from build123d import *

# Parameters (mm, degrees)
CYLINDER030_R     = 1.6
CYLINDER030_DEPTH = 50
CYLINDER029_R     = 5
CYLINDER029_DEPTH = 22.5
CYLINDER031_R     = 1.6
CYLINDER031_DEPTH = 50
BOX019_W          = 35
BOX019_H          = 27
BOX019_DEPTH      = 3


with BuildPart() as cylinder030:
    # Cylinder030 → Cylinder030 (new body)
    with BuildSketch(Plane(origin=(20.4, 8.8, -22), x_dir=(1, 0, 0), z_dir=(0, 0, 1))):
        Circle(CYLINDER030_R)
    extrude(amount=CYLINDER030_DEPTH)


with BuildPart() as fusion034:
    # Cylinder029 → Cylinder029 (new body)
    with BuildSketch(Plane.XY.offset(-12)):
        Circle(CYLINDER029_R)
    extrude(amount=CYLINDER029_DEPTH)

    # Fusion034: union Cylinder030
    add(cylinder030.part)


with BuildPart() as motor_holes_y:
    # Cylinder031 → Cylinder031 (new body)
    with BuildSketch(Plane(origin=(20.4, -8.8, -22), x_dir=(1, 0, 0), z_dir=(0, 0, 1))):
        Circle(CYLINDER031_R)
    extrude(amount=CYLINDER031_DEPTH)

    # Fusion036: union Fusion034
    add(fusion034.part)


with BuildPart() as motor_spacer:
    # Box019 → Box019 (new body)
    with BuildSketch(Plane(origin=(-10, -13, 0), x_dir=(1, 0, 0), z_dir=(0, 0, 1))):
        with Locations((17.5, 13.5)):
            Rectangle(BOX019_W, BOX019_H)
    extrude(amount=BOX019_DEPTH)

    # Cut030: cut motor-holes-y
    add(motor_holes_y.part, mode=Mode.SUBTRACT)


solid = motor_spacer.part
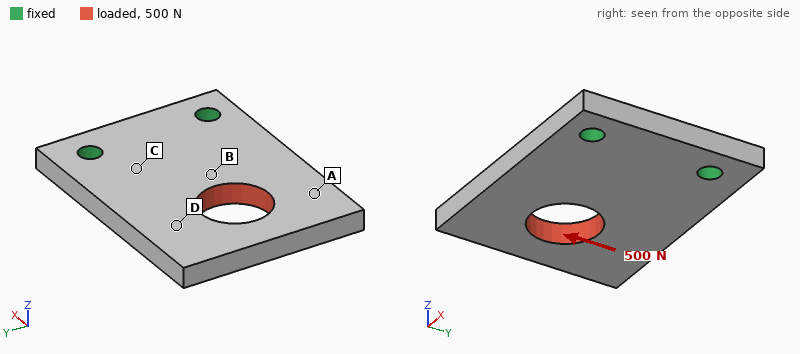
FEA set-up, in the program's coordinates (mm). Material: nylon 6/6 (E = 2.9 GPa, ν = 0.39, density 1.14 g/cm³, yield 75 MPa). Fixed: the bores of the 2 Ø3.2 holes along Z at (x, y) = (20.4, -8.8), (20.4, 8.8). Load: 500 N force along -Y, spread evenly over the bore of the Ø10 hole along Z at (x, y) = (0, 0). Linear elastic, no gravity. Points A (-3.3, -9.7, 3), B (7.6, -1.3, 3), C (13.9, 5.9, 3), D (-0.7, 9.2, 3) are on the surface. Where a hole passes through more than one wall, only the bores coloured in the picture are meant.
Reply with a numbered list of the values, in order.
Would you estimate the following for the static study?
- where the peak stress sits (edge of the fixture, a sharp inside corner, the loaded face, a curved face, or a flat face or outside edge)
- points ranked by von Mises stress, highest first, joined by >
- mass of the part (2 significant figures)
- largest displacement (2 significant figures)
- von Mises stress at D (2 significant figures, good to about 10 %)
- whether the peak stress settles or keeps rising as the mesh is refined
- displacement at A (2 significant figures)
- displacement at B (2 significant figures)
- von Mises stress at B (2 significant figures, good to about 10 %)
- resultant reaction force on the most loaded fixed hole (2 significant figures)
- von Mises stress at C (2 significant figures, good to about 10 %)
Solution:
1. edge of the fixture
2. B > C > D > A
3. 2.9 g
4. 0.46 mm
5. 11 MPa
6. keeps rising
7. 0.36 mm
8. 0.15 mm
9. 23 MPa
10. 580 N
11. 16 MPa
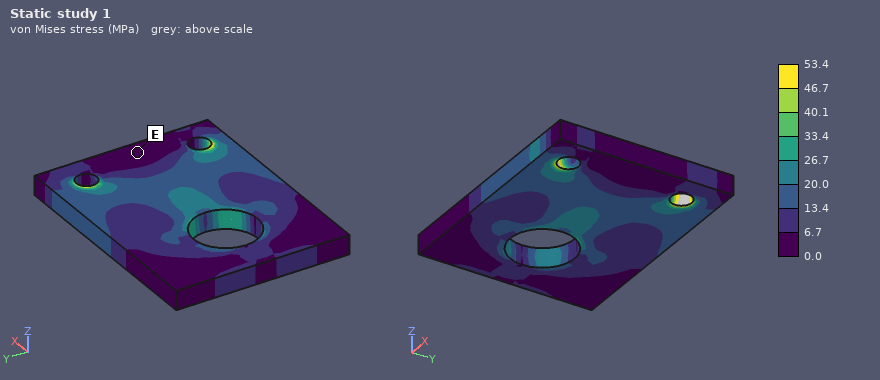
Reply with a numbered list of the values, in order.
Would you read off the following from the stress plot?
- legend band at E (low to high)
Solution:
1. 0.0 to 6.7 MPa
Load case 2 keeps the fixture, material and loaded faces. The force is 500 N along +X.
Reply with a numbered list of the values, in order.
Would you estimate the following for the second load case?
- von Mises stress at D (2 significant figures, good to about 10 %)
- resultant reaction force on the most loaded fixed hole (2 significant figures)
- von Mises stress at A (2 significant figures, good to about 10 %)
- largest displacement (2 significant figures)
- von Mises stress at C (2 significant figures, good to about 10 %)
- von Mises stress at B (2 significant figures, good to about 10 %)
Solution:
1. 4.3 MPa
2. 250 N
3. 2.1 MPa
4. 0.10 mm
5. 7.2 MPa
6. 6.0 MPa
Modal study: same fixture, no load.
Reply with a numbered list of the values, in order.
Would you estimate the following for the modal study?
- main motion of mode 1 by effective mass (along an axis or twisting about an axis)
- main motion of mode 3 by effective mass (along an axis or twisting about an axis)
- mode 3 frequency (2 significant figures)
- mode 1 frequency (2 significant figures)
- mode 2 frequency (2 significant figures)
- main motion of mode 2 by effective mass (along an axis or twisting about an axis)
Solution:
1. along Z
2. along Z
3. 4700 Hz
4. 890 Hz
5. 2000 Hz
6. twisting about X
